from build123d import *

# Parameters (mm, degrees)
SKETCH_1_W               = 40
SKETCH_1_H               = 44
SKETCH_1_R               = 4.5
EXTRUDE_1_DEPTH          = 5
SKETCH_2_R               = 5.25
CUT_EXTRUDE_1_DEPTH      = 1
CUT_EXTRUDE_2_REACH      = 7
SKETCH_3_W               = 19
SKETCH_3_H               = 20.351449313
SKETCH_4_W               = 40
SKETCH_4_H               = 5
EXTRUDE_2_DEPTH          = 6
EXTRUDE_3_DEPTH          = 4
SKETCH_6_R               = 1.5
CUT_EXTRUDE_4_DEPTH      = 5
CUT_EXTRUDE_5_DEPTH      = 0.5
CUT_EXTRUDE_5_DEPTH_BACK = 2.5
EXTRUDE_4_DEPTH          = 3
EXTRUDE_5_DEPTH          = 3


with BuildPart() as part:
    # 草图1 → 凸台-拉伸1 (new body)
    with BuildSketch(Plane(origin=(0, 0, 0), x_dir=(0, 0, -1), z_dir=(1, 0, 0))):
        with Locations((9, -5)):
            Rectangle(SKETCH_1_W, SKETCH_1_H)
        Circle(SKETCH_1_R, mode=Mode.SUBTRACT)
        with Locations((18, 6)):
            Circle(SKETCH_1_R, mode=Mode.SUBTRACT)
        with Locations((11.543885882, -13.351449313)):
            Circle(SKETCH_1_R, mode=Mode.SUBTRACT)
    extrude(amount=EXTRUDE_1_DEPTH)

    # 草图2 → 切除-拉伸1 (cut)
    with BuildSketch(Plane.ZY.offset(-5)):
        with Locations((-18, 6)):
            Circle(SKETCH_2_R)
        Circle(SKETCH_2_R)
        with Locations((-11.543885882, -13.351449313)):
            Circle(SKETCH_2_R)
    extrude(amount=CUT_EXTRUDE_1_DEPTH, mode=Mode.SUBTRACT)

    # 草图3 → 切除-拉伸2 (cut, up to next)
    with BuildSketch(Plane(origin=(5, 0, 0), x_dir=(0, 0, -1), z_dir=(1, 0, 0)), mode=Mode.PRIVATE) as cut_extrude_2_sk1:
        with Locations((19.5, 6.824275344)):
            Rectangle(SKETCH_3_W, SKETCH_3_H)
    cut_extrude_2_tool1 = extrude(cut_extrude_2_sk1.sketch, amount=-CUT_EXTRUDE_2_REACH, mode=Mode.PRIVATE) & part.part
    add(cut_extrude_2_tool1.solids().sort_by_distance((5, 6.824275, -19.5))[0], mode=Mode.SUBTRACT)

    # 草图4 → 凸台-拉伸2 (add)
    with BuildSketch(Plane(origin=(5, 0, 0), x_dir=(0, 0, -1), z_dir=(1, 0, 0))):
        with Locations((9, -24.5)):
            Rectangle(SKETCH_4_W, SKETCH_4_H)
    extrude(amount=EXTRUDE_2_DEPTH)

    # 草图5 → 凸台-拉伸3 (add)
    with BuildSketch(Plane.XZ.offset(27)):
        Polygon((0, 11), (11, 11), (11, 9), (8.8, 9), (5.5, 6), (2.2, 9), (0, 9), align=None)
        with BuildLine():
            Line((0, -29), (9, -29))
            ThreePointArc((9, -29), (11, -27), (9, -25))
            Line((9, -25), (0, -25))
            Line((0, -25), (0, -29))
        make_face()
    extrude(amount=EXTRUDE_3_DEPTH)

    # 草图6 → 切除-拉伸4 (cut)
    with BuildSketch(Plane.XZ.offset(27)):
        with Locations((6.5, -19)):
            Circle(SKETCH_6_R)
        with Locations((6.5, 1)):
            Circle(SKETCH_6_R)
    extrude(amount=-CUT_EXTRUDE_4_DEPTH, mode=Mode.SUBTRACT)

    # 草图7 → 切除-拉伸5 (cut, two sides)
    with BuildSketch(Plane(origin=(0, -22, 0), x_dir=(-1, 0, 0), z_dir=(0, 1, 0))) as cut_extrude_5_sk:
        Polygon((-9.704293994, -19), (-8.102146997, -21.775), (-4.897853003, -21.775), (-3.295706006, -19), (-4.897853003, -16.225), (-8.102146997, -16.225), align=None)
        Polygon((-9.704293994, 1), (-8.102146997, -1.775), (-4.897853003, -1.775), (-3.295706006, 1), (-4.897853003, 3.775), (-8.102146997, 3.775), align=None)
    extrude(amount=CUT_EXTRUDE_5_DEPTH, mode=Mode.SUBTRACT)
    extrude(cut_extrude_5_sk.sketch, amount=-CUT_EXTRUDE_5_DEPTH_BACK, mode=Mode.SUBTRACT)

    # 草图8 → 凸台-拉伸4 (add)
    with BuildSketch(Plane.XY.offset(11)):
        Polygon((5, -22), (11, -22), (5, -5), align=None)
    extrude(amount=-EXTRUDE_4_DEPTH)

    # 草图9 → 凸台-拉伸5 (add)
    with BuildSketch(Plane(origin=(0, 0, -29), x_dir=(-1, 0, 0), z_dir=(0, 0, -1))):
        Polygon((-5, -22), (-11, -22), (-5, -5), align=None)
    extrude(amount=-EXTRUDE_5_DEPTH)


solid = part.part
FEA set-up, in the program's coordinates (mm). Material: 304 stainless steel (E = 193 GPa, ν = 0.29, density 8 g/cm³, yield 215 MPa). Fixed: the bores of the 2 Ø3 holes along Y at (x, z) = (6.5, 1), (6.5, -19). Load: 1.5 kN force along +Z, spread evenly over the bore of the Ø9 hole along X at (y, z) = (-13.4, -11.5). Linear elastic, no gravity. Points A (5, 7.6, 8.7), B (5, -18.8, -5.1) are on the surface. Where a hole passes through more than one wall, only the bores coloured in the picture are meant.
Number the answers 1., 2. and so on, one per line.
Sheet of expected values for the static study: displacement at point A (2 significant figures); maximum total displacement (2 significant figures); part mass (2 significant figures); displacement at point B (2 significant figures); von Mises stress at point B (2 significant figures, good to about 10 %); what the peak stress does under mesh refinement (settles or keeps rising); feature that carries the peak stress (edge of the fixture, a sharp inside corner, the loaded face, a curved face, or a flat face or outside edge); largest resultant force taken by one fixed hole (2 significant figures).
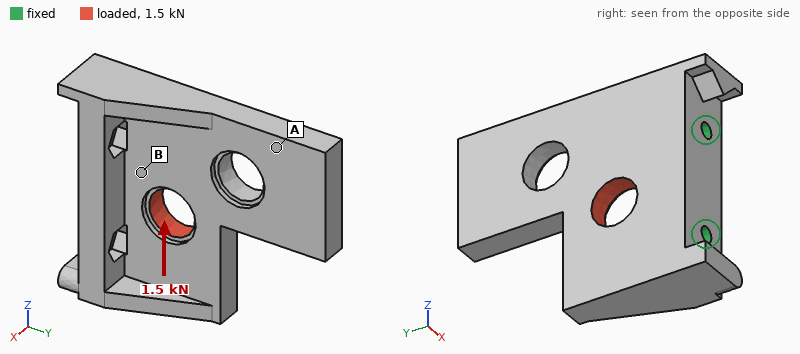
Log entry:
1. 15 µm
2. 18 µm
3. 63 g
4. 3.4 µm
5. 25 MPa
6. keeps rising
7. edge of the fixture
8. 1.2 kN
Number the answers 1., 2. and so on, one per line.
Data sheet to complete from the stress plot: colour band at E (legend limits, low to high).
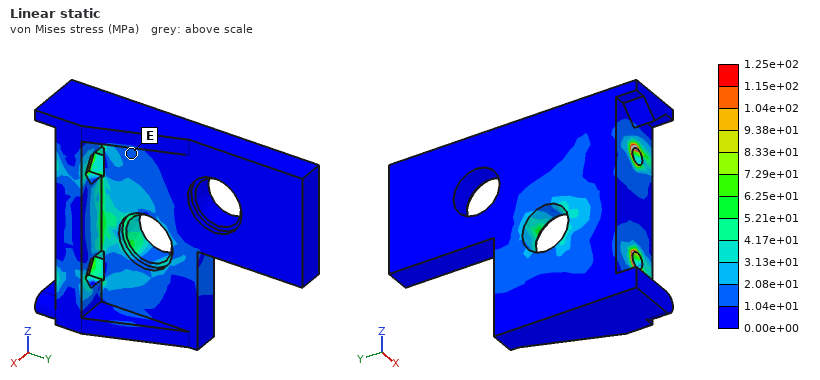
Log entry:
1. 1.04e+01 to 2.08e+01 MPa
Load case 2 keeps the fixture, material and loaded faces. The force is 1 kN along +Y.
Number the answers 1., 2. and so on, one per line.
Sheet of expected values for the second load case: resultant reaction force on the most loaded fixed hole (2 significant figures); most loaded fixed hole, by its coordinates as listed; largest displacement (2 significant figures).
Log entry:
1. 620 N
2. (6.5, -19)
3. 31 µm
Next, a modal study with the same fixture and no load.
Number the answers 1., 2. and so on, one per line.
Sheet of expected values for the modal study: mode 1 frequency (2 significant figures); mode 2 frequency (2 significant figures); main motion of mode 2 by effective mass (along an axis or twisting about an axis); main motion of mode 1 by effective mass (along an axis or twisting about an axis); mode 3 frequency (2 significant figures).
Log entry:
1. 1900 Hz
2. 5600 Hz
3. along Z
4. along X
5. 7400 Hz
